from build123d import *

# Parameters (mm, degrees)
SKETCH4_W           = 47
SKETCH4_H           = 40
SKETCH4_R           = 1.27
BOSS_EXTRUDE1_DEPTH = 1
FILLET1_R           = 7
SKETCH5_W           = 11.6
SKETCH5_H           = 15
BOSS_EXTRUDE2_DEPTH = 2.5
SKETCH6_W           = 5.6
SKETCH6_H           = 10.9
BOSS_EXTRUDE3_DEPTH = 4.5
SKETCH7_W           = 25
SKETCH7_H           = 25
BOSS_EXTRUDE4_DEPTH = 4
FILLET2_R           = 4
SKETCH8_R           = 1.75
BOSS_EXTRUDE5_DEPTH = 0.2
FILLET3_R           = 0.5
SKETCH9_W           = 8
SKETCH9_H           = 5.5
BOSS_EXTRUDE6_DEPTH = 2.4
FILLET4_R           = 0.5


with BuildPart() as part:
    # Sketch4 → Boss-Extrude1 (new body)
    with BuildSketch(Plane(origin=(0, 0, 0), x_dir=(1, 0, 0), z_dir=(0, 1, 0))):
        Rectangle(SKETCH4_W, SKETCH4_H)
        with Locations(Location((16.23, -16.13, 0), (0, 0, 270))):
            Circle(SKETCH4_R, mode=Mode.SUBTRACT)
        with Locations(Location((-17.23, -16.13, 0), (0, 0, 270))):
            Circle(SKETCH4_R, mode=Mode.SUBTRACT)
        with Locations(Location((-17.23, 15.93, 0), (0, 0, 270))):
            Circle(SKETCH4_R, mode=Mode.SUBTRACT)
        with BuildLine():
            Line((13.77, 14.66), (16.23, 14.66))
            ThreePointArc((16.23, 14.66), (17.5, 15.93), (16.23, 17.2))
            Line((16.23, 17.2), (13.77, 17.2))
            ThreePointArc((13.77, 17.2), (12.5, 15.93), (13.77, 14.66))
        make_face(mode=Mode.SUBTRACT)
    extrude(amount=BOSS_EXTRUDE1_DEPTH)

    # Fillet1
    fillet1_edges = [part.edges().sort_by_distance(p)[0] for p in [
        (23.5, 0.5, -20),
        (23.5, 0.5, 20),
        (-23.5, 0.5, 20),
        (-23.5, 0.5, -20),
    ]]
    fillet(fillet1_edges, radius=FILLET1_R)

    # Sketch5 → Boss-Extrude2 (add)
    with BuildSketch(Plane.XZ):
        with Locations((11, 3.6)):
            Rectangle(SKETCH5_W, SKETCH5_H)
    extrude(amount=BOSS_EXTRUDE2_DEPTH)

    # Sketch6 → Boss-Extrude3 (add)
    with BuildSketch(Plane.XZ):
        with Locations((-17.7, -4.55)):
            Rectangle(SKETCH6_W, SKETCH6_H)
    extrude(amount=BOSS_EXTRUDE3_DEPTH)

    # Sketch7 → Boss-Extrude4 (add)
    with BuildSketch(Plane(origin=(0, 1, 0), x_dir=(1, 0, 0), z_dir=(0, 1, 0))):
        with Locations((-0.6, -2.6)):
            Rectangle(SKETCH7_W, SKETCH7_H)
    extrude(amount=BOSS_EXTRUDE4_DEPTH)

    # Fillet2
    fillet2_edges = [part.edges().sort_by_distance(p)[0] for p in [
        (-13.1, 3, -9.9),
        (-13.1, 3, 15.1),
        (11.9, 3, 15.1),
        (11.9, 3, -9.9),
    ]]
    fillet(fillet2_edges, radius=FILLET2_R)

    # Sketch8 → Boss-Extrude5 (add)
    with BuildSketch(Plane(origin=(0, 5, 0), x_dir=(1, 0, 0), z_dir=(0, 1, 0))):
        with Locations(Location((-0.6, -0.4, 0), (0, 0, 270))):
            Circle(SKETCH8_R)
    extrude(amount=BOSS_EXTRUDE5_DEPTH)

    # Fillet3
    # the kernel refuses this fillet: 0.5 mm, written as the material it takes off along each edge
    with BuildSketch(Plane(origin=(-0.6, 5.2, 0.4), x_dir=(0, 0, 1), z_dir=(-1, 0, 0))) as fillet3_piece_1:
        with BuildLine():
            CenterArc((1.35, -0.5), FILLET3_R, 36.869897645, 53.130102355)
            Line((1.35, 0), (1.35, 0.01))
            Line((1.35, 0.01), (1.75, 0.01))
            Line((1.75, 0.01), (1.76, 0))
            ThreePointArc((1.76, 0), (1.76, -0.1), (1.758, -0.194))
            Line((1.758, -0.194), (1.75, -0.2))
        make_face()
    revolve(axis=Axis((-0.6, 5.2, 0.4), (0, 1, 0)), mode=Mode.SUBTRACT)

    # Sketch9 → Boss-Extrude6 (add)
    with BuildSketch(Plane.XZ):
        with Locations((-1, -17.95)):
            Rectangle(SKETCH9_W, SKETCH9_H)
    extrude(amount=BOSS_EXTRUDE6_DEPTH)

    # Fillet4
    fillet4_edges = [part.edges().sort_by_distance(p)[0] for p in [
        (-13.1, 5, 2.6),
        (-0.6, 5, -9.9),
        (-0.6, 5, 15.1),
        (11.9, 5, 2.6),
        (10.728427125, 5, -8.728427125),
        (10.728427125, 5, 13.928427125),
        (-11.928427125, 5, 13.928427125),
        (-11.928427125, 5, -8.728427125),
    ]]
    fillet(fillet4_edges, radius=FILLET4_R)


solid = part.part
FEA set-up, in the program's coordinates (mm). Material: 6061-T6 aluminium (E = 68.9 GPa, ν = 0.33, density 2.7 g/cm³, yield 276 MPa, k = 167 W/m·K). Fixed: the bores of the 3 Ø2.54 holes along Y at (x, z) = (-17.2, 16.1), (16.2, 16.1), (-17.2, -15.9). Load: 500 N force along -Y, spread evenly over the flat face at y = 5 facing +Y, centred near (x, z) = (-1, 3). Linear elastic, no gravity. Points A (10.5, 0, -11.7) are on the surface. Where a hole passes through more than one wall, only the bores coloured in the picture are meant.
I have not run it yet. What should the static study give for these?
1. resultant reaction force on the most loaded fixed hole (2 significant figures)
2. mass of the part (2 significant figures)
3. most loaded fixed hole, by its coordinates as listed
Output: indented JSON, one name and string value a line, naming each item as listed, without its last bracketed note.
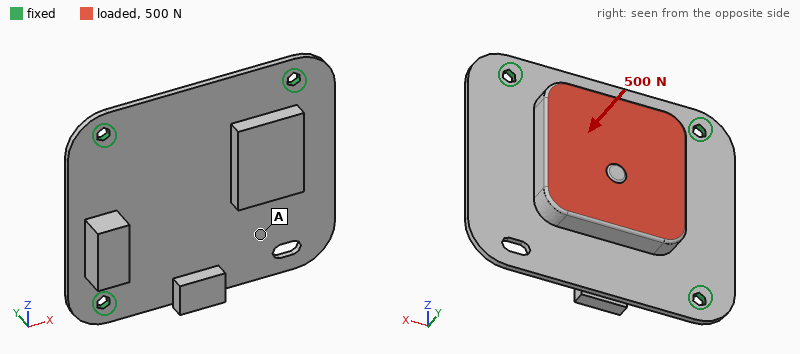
{
  "resultant reaction force on the most loaded fixed hole": "290 N",
  "mass of the part": "14 g",
  "most loaded fixed hole, by its coordinates as listed": "(16.2, 16.1)"
}
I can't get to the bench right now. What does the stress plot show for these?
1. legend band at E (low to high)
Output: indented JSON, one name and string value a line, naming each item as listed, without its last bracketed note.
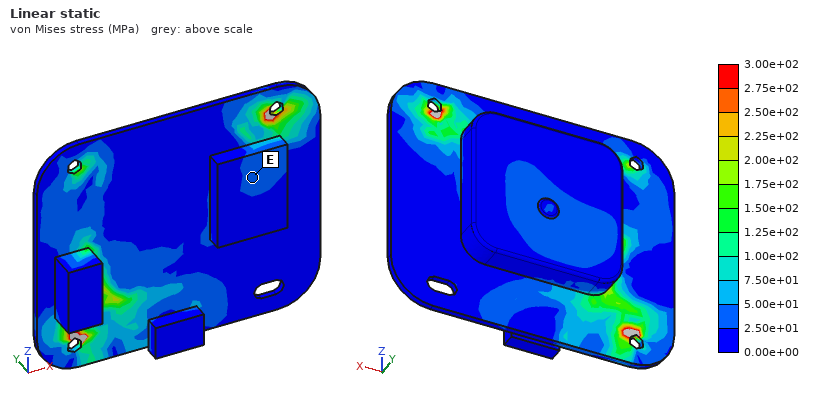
{
  "legend band at E": "2.50e+01 to 5.00e+01 MPa"
}
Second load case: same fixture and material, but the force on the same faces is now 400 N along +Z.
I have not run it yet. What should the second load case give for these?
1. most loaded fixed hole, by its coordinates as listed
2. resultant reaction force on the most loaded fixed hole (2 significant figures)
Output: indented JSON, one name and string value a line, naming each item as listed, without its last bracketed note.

{
  "most loaded fixed hole, by its coordinates as listed": "(-17.2, 16.1)",
  "resultant reaction force on the most loaded fixed hole": "190 N"
}
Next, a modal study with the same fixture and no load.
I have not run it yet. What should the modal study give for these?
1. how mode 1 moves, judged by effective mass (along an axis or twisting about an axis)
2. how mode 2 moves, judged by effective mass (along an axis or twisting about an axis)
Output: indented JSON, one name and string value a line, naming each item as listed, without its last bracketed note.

{
  "how mode 1 moves, judged by effective mass": "along Y",
  "how mode 2 moves, judged by effective mass": "along Y"
}
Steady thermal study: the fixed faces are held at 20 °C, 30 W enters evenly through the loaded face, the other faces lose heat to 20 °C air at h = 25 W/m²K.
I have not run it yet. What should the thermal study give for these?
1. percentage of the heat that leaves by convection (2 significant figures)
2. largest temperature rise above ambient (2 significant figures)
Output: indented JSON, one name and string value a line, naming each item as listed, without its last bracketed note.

{
  "percentage of the heat that leaves by convection": "8.8 %",
  "largest temperature rise above ambient": "37 K"
}
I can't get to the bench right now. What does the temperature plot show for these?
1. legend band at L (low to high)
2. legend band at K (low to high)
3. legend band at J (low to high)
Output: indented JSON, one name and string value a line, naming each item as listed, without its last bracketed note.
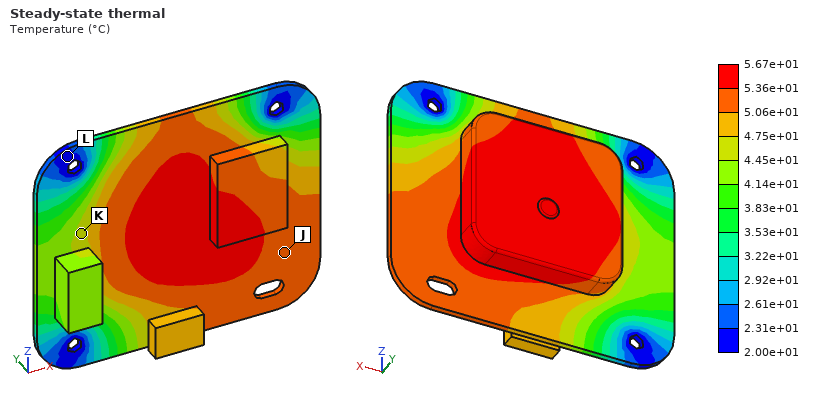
{
  "legend band at L": "2.00e+01 to 2.31e+01 °C",
  "legend band at K": "4.45e+01 to 4.75e+01 °C",
  "legend band at J": "5.06e+01 to 5.36e+01 °C"
}
